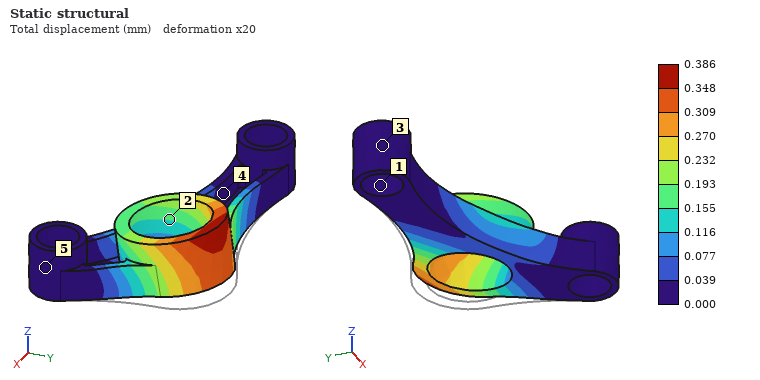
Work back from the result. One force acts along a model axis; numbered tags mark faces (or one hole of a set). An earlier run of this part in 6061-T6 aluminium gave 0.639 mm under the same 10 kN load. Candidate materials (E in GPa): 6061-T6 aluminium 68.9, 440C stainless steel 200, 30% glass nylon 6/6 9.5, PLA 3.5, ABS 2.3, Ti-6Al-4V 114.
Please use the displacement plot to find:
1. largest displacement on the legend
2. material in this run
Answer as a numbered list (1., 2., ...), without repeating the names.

1. 0.386 mm
2. Ti-6Al-4V
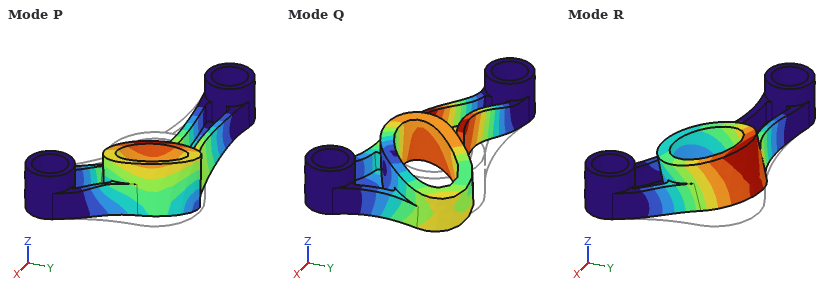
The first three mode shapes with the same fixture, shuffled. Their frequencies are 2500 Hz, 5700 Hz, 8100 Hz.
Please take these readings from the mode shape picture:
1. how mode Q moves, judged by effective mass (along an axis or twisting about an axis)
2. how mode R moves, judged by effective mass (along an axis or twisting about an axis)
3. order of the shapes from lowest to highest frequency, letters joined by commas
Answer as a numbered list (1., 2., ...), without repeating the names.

1. along Y
2. along Z
3. R, P, Q
